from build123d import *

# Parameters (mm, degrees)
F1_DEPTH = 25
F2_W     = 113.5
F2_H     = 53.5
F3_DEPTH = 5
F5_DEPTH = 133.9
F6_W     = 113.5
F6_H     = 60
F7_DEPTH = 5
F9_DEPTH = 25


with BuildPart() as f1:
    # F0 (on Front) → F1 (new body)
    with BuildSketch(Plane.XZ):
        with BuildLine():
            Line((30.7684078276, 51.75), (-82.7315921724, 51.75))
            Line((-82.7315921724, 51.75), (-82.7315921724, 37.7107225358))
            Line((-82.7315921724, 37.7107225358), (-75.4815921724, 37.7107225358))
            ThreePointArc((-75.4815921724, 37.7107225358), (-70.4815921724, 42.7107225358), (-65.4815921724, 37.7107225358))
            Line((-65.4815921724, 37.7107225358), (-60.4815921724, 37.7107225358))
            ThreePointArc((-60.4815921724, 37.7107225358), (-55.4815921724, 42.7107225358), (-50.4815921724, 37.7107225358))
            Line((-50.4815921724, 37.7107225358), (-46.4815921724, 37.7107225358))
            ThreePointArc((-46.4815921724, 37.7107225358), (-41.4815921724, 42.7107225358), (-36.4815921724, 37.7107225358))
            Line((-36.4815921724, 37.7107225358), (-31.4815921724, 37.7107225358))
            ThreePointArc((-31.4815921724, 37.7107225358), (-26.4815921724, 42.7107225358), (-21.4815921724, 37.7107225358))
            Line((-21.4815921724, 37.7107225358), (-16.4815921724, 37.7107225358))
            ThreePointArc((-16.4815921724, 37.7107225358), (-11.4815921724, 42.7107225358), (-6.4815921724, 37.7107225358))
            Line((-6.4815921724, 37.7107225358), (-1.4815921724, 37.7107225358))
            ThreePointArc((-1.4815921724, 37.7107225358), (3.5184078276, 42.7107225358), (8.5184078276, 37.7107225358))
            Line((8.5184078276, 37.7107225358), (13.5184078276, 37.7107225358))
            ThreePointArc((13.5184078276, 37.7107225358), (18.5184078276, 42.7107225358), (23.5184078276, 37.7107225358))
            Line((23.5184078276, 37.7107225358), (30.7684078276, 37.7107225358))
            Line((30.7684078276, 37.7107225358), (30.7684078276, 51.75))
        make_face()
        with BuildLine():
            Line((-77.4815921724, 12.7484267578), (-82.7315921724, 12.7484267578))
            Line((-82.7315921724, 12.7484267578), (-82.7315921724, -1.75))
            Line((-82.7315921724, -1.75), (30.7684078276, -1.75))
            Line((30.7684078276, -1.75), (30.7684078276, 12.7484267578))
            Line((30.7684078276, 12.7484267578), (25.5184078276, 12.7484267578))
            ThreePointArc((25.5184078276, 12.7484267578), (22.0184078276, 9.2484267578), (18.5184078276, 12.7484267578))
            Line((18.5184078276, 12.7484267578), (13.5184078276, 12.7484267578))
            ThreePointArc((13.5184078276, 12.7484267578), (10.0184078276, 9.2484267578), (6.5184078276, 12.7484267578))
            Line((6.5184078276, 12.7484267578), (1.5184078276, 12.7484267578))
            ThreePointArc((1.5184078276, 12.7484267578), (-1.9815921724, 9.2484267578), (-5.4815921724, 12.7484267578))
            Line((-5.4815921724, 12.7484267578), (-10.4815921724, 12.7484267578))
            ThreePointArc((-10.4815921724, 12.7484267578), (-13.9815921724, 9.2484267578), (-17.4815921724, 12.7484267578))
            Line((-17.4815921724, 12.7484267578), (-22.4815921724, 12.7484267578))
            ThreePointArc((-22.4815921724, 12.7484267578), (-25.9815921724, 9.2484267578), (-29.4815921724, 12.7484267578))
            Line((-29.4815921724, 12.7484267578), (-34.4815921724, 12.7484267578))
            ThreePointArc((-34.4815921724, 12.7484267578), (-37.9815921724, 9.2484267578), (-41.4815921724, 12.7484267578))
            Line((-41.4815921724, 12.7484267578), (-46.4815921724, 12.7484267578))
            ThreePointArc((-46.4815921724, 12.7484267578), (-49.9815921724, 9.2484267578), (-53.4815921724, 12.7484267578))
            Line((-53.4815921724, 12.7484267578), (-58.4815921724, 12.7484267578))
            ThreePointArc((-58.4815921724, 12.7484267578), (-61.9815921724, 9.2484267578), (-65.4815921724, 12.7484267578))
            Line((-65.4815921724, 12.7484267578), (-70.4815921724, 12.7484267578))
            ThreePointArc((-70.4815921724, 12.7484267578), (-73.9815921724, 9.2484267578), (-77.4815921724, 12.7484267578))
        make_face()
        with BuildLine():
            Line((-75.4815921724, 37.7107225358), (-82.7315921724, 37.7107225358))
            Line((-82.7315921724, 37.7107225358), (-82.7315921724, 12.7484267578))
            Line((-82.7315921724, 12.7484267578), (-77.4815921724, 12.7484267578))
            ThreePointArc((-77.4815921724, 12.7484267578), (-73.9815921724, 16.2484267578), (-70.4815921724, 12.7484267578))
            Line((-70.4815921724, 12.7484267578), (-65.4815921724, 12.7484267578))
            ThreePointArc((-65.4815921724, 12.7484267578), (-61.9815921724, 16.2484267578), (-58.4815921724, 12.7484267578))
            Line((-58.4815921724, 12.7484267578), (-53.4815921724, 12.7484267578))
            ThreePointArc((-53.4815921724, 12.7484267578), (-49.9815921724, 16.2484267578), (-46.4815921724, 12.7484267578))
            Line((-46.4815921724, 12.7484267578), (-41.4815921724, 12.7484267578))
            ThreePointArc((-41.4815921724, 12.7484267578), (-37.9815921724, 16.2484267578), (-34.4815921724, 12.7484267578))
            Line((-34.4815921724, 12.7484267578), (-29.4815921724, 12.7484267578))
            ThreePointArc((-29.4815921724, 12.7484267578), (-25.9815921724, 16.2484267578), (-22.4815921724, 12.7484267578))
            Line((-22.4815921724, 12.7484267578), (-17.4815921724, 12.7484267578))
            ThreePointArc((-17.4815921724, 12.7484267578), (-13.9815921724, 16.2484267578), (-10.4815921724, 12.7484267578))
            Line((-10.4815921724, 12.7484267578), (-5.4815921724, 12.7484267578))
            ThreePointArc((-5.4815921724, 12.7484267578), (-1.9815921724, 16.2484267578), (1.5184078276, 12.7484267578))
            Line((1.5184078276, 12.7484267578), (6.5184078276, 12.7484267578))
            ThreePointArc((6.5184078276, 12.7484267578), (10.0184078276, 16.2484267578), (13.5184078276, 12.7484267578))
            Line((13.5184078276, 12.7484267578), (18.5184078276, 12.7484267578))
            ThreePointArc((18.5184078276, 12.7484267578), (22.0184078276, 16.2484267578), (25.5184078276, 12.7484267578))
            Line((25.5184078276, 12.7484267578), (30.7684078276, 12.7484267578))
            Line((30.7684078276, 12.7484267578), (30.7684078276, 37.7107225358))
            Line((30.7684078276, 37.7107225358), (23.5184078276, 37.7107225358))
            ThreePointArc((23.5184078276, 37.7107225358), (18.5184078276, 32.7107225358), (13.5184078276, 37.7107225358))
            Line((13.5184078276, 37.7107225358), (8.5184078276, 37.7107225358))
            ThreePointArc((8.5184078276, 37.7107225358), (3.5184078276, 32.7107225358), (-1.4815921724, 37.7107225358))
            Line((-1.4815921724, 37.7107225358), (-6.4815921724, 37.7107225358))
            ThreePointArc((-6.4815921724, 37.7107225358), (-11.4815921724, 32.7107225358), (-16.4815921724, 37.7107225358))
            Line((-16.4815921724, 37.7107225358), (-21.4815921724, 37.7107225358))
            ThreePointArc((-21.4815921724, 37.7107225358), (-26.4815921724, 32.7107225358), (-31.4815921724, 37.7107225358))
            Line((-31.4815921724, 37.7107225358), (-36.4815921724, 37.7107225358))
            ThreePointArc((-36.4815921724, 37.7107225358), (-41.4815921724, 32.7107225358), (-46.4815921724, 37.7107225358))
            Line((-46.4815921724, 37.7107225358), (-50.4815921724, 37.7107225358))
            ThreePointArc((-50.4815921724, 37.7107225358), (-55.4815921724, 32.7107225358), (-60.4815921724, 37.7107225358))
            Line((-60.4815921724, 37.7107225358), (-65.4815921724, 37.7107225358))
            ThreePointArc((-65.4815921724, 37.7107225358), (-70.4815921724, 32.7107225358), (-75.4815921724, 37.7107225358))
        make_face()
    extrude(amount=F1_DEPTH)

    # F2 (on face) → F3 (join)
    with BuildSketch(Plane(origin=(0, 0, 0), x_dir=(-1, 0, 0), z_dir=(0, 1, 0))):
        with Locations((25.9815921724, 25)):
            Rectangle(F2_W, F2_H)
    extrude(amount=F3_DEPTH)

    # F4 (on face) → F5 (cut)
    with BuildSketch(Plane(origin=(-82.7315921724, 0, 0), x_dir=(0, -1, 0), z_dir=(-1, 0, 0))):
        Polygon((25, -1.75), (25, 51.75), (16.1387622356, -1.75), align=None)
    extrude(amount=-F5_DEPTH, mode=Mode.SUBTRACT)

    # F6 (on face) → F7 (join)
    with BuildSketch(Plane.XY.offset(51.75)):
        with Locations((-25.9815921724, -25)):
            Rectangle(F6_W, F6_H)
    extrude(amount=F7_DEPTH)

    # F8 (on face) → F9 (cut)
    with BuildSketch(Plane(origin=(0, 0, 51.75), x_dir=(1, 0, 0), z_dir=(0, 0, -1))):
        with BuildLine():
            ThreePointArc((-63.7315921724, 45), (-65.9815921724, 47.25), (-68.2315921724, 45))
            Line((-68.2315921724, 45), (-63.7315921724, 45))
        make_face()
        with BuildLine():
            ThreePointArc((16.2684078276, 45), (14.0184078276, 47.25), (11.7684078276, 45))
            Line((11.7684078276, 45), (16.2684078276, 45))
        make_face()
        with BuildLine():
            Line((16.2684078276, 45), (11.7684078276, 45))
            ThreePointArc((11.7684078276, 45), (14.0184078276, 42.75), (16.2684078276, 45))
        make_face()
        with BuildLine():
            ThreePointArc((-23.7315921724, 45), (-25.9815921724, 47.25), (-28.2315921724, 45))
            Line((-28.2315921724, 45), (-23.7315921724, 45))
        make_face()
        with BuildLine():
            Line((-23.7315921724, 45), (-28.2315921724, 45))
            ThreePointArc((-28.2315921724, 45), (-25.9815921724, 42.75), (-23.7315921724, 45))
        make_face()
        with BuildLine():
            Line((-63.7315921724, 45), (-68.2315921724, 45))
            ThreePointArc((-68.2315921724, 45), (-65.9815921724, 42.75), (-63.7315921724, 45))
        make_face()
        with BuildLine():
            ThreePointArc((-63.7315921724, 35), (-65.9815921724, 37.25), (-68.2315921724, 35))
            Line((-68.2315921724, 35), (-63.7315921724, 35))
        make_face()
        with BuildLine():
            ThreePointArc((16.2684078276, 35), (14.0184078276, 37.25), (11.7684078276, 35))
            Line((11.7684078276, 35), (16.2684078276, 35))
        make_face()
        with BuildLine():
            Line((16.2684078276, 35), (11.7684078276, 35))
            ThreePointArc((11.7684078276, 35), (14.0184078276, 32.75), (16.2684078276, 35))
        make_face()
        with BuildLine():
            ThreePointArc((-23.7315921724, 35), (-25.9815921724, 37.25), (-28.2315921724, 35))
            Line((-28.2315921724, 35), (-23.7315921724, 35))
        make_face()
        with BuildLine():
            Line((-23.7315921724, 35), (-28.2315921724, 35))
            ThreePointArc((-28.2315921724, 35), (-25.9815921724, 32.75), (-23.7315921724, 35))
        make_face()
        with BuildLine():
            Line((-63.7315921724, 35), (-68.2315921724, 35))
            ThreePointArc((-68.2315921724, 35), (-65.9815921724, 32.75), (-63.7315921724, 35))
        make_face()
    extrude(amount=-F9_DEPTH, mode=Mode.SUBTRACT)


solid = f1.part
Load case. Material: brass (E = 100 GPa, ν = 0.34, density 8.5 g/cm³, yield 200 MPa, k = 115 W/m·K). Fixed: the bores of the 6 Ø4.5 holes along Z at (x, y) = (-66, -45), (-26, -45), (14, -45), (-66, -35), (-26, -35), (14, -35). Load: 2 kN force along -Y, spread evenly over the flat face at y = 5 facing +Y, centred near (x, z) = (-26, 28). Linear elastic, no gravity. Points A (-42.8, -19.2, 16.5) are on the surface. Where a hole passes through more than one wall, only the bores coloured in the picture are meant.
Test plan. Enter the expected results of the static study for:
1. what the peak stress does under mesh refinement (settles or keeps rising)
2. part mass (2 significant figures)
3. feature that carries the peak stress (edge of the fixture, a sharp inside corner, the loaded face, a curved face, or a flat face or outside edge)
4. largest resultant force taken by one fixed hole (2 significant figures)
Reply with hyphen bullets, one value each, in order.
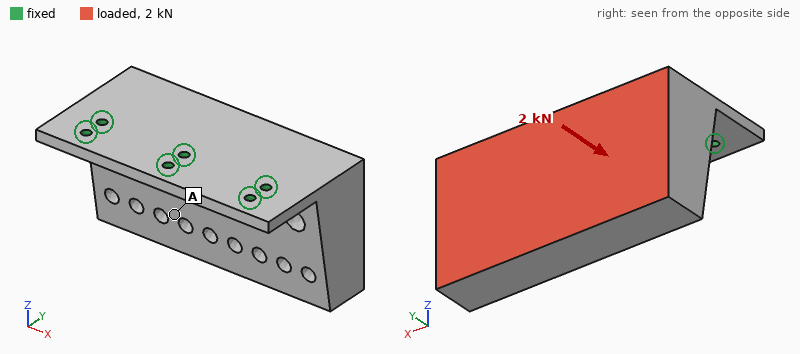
- keeps rising
- 1.4 kg
- edge of the fixture
- 870 N
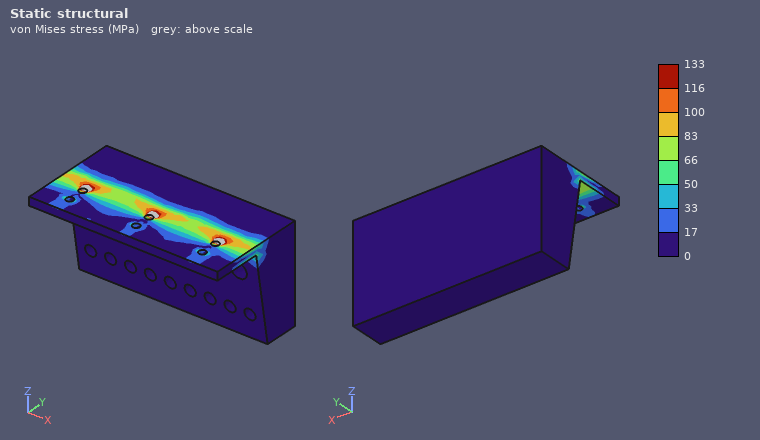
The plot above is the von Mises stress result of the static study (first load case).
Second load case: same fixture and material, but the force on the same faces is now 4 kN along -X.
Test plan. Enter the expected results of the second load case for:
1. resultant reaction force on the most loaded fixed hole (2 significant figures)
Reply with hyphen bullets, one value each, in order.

- 2.3 kN
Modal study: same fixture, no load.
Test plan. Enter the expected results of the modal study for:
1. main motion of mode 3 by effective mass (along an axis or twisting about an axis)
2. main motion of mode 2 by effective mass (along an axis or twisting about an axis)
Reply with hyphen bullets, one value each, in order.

- along Z
- along X
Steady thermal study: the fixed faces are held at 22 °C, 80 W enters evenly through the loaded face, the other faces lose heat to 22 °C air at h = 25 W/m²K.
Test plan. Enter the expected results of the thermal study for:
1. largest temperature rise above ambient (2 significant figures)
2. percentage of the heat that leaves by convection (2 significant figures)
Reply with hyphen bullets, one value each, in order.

- 28 K
- 19 %
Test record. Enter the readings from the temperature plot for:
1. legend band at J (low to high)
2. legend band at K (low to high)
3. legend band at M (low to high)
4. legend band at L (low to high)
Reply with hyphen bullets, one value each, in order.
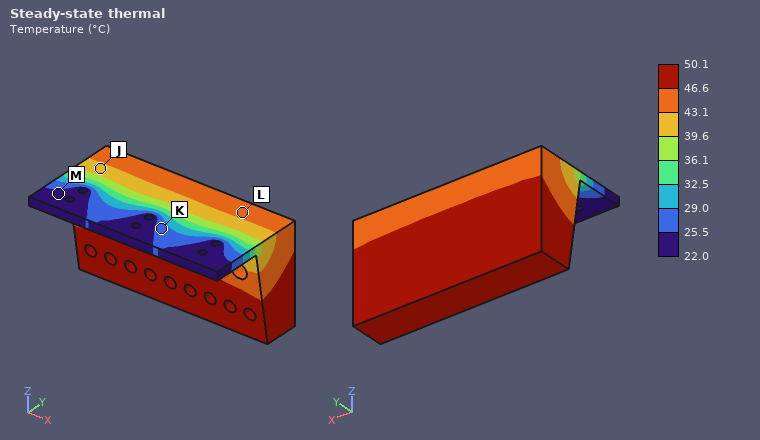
- 39.6 to 43.1 °C
- 25.5 to 29.0 °C
- 22.0 to 25.5 °C
- 43.1 to 46.6 °C
